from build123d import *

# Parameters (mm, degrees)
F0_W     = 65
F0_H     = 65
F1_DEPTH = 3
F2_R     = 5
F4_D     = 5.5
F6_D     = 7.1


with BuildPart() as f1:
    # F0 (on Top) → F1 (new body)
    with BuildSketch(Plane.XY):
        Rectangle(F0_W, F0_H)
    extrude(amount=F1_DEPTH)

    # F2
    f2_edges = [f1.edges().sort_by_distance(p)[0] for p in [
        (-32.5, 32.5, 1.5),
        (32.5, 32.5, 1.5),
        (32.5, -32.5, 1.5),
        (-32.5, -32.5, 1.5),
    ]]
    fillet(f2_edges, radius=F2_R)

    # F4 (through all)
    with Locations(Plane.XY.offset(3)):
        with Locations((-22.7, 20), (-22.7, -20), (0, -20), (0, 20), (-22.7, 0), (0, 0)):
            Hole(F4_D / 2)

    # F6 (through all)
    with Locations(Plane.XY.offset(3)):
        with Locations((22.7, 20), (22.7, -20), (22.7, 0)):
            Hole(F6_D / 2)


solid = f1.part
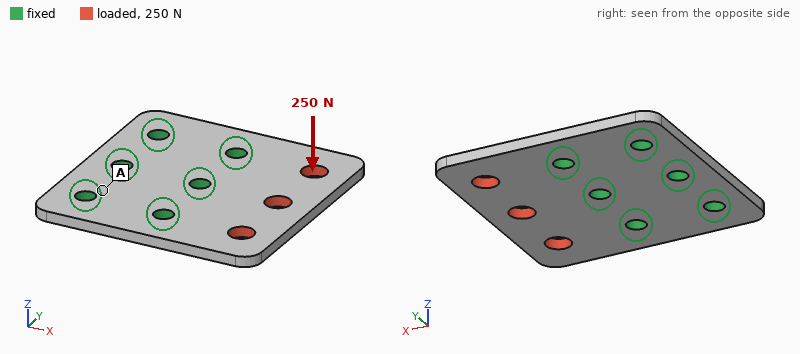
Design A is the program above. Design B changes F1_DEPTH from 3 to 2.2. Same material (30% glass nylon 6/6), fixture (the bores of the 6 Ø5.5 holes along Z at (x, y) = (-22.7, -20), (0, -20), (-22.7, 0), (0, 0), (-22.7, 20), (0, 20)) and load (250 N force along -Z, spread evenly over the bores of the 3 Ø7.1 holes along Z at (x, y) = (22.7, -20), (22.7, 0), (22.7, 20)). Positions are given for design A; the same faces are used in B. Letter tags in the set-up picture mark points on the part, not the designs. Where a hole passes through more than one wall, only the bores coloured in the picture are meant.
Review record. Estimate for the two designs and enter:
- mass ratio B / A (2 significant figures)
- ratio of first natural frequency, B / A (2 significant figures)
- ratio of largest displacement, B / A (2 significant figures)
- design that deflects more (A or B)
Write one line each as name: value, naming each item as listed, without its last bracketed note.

mass ratio B / A: 0.73
ratio of first natural frequency, B / A: 0.74
ratio of largest displacement, B / A: 2.5
design that deflects more: B
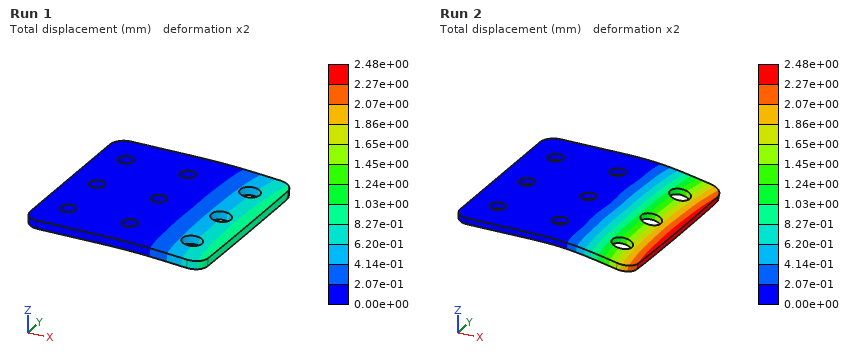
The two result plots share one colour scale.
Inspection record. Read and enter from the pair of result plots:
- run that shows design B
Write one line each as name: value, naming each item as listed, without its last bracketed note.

run that shows design B: Run 2
